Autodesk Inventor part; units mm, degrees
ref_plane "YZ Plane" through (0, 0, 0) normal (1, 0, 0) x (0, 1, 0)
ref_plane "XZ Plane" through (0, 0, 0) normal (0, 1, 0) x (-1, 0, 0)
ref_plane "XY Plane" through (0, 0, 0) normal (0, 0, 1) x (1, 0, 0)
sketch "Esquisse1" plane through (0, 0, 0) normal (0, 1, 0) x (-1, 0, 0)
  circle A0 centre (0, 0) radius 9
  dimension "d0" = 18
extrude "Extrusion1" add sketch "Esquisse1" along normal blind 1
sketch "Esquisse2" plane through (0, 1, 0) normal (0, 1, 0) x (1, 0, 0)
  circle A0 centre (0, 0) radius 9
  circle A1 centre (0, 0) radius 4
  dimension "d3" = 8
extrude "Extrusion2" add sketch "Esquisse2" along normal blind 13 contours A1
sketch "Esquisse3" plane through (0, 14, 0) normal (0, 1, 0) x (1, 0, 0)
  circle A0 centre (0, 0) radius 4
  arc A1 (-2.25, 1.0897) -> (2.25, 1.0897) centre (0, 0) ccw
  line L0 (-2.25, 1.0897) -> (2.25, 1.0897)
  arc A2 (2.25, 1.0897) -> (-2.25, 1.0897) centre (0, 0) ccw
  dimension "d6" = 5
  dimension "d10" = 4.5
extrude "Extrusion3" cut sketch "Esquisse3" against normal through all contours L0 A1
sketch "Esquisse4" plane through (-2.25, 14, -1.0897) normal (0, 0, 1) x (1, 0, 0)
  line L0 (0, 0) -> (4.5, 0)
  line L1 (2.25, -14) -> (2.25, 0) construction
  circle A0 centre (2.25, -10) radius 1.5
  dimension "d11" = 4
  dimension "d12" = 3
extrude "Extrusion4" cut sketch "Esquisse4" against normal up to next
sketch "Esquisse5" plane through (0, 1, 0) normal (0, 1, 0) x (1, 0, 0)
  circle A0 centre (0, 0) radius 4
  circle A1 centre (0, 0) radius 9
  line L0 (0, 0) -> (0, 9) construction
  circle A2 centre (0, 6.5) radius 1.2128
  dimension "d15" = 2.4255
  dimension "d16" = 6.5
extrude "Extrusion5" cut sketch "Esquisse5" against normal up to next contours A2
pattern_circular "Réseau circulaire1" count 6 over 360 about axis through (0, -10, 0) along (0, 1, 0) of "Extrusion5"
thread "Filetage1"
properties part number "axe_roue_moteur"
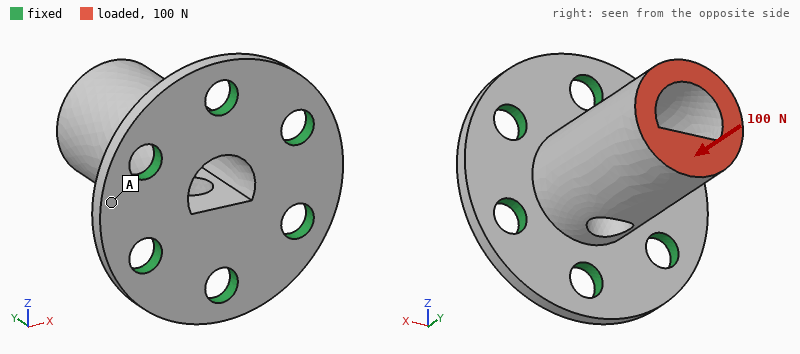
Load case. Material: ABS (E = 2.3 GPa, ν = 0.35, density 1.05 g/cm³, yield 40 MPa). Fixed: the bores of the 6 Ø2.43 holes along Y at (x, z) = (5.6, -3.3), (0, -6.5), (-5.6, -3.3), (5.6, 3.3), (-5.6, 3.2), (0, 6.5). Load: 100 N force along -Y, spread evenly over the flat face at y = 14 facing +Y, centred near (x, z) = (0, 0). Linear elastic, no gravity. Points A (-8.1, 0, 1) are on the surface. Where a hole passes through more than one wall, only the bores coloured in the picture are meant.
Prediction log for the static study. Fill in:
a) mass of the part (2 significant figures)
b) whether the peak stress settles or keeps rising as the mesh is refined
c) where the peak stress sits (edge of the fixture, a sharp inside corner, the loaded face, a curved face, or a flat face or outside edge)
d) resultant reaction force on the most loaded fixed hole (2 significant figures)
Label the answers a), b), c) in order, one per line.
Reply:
a) 0.68 g
b) keeps rising
c) edge of the fixture
d) 20 N
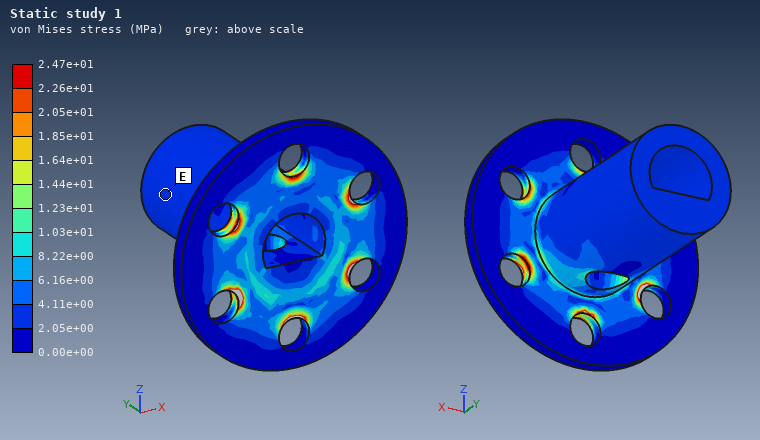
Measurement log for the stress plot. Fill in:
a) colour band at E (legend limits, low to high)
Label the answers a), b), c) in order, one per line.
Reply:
a) 2.05e+00 to 4.11e+00 MPa
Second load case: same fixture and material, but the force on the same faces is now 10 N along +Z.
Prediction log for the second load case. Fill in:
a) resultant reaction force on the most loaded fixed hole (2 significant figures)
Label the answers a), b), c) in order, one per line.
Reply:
a) 10 N
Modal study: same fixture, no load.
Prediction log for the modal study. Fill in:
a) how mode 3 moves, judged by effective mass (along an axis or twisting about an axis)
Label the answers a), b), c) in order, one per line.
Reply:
a) along Y
